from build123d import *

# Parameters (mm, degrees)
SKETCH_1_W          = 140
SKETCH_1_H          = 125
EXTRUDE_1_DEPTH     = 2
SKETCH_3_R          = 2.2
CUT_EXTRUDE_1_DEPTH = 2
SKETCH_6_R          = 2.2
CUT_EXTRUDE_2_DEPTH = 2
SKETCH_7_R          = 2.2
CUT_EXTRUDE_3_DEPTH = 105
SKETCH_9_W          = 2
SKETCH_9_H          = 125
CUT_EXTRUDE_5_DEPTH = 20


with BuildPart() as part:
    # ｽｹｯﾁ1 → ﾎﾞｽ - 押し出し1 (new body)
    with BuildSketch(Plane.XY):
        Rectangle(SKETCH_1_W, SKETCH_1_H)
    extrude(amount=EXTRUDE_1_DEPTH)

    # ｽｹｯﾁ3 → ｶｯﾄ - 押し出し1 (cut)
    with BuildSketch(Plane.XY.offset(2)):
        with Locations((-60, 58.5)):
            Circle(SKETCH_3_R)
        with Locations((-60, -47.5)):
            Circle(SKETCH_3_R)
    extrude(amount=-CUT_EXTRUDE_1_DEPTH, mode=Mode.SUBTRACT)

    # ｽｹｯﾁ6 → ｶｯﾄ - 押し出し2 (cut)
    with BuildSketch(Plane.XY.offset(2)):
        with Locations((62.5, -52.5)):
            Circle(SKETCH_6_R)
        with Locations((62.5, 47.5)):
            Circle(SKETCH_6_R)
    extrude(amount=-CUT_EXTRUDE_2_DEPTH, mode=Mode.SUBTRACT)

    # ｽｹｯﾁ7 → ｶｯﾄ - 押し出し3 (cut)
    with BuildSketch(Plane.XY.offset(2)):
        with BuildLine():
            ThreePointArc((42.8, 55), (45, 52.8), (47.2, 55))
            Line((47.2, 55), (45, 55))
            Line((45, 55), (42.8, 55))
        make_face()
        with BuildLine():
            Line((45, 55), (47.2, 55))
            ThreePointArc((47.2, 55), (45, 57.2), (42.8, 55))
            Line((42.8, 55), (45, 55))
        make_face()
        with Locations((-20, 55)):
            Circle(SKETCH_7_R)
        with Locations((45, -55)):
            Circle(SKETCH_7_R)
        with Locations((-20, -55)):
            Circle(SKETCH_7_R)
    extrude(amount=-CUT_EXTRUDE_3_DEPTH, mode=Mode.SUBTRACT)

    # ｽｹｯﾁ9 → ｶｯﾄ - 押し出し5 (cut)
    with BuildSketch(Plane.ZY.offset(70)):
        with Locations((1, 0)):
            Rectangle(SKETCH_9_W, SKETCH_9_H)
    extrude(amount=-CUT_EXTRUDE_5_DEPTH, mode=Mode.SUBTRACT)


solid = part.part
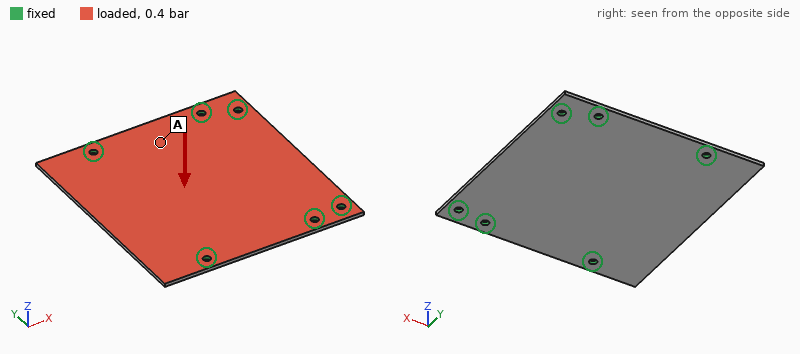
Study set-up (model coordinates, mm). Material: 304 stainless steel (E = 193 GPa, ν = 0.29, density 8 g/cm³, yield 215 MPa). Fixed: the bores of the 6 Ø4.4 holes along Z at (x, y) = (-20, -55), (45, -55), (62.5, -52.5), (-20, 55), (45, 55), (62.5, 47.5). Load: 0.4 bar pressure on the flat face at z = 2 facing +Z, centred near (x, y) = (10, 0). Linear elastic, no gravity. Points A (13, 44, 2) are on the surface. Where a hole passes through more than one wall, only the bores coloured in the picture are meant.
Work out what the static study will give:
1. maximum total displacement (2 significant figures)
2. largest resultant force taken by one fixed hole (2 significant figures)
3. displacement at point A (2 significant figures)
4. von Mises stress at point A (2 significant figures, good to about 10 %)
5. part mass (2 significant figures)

0.21 mm
160 N
0.046 mm
18 MPa
240 g
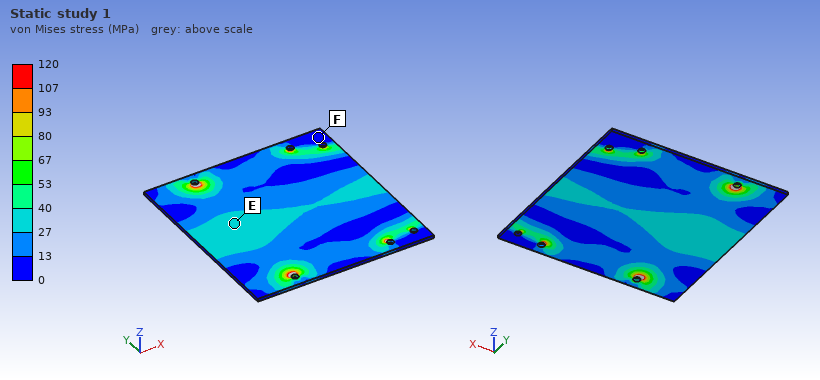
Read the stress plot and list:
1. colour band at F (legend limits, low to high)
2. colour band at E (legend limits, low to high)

0 to 13 MPa
27 to 40 MPa
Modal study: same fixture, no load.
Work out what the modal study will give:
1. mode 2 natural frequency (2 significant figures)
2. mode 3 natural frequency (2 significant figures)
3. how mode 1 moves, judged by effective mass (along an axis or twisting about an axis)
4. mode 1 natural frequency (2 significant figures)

920 Hz
1400 Hz
along Z
720 Hz
